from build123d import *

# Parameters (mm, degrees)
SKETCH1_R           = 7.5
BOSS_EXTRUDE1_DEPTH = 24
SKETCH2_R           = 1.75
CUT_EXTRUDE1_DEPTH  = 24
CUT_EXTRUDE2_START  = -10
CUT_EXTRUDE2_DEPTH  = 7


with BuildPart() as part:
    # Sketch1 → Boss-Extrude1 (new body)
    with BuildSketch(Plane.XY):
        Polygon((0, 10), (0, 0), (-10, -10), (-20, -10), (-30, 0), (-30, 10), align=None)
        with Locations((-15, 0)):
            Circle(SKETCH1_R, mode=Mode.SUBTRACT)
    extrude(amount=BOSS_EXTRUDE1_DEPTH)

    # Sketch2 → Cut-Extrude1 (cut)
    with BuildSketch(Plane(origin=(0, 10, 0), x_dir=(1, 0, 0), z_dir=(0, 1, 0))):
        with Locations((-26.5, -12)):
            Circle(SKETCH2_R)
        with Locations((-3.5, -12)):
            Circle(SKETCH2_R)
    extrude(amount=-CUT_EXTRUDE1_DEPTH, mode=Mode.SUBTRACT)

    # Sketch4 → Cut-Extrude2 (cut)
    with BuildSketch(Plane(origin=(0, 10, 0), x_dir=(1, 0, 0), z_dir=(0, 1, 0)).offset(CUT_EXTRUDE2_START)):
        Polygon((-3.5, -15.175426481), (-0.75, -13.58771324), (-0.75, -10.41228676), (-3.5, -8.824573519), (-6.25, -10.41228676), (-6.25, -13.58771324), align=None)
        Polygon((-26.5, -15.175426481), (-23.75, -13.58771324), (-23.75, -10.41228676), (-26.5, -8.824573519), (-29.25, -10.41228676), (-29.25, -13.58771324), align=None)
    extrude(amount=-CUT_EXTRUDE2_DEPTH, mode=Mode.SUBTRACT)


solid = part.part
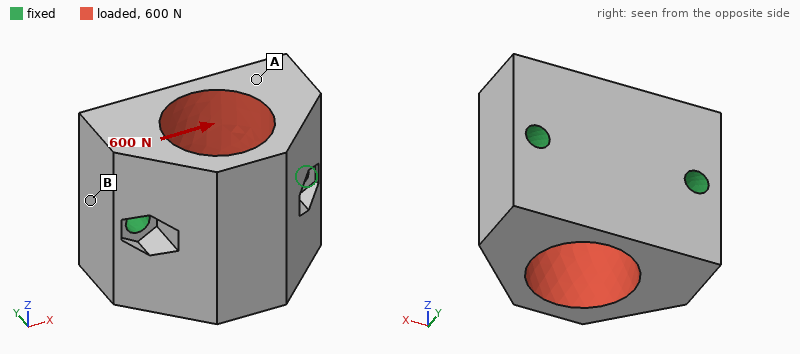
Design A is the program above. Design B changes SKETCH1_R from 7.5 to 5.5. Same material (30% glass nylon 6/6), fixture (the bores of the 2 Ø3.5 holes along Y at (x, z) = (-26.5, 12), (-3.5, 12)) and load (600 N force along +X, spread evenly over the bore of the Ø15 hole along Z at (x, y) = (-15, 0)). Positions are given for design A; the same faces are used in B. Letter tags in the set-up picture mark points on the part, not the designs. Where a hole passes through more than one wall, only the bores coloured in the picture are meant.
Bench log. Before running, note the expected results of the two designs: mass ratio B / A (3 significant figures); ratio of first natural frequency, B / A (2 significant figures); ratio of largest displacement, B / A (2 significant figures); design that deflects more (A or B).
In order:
1.27
0.93
0.48
A
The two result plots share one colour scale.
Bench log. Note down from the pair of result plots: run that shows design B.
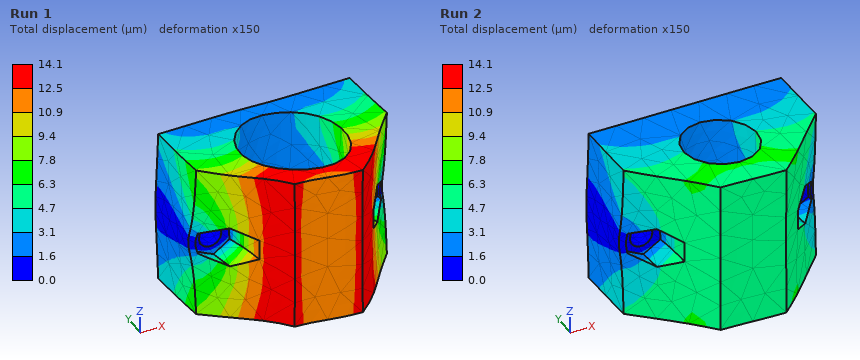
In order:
Run 2
